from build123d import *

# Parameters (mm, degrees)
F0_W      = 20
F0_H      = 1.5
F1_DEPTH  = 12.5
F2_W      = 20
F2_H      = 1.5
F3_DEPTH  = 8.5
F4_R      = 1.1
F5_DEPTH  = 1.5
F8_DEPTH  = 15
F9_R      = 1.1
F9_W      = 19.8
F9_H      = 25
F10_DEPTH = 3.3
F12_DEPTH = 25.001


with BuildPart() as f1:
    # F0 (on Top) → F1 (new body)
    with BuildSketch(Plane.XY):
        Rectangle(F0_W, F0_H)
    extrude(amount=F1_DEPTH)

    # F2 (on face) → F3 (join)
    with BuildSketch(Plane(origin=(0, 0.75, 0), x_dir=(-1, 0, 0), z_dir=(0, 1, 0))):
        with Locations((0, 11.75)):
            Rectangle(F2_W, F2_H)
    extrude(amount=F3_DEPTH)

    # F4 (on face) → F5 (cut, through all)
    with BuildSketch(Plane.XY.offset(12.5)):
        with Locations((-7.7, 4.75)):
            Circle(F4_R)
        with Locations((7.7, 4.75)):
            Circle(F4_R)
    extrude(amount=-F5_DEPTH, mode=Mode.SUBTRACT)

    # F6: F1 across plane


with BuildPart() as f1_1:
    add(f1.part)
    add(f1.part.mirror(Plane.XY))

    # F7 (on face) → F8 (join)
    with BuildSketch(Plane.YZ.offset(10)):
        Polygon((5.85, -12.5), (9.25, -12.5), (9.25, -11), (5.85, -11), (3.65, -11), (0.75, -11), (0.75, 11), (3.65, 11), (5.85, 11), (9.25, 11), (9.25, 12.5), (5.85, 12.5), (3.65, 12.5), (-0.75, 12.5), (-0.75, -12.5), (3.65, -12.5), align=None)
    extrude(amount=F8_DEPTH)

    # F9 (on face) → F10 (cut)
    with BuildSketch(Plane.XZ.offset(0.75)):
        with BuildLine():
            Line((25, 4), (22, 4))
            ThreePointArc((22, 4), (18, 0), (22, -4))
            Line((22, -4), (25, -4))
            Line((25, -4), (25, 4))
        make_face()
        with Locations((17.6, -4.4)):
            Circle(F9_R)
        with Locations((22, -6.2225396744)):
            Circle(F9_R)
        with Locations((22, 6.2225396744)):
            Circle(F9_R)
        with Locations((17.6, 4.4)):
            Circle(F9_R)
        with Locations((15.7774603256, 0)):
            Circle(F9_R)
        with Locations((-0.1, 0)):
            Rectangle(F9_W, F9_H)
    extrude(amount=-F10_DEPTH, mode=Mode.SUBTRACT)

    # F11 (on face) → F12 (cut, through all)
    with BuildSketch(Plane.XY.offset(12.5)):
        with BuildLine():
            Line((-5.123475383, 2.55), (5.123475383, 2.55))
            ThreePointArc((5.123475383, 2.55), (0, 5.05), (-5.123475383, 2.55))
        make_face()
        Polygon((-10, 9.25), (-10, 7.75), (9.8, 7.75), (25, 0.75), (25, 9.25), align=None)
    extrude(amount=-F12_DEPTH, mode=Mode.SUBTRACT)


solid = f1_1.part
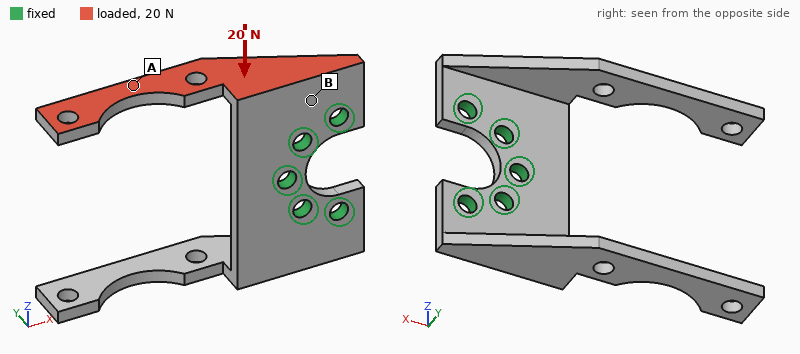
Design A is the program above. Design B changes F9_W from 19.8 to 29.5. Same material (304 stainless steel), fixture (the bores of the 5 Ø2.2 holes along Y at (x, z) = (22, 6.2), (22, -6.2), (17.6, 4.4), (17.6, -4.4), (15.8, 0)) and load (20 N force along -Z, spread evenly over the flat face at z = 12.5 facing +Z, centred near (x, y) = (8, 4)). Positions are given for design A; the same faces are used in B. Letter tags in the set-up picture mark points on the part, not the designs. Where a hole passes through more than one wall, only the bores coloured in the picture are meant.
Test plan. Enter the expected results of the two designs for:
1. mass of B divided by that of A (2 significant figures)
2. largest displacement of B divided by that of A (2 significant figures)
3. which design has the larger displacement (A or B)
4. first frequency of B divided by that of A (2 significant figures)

0.76
2.4
B
0.68
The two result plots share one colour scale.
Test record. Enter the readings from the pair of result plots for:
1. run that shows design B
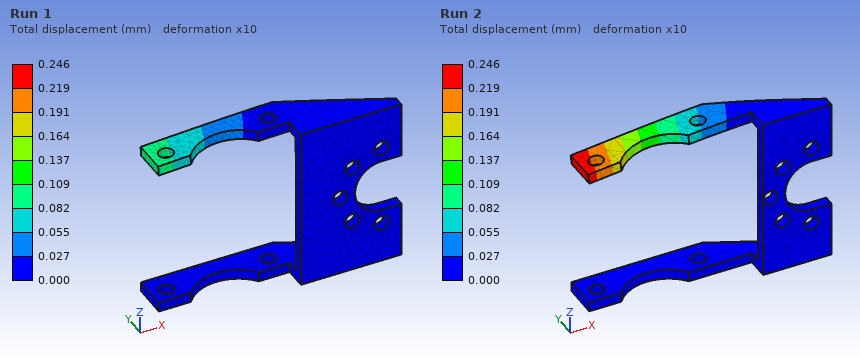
Run 2
